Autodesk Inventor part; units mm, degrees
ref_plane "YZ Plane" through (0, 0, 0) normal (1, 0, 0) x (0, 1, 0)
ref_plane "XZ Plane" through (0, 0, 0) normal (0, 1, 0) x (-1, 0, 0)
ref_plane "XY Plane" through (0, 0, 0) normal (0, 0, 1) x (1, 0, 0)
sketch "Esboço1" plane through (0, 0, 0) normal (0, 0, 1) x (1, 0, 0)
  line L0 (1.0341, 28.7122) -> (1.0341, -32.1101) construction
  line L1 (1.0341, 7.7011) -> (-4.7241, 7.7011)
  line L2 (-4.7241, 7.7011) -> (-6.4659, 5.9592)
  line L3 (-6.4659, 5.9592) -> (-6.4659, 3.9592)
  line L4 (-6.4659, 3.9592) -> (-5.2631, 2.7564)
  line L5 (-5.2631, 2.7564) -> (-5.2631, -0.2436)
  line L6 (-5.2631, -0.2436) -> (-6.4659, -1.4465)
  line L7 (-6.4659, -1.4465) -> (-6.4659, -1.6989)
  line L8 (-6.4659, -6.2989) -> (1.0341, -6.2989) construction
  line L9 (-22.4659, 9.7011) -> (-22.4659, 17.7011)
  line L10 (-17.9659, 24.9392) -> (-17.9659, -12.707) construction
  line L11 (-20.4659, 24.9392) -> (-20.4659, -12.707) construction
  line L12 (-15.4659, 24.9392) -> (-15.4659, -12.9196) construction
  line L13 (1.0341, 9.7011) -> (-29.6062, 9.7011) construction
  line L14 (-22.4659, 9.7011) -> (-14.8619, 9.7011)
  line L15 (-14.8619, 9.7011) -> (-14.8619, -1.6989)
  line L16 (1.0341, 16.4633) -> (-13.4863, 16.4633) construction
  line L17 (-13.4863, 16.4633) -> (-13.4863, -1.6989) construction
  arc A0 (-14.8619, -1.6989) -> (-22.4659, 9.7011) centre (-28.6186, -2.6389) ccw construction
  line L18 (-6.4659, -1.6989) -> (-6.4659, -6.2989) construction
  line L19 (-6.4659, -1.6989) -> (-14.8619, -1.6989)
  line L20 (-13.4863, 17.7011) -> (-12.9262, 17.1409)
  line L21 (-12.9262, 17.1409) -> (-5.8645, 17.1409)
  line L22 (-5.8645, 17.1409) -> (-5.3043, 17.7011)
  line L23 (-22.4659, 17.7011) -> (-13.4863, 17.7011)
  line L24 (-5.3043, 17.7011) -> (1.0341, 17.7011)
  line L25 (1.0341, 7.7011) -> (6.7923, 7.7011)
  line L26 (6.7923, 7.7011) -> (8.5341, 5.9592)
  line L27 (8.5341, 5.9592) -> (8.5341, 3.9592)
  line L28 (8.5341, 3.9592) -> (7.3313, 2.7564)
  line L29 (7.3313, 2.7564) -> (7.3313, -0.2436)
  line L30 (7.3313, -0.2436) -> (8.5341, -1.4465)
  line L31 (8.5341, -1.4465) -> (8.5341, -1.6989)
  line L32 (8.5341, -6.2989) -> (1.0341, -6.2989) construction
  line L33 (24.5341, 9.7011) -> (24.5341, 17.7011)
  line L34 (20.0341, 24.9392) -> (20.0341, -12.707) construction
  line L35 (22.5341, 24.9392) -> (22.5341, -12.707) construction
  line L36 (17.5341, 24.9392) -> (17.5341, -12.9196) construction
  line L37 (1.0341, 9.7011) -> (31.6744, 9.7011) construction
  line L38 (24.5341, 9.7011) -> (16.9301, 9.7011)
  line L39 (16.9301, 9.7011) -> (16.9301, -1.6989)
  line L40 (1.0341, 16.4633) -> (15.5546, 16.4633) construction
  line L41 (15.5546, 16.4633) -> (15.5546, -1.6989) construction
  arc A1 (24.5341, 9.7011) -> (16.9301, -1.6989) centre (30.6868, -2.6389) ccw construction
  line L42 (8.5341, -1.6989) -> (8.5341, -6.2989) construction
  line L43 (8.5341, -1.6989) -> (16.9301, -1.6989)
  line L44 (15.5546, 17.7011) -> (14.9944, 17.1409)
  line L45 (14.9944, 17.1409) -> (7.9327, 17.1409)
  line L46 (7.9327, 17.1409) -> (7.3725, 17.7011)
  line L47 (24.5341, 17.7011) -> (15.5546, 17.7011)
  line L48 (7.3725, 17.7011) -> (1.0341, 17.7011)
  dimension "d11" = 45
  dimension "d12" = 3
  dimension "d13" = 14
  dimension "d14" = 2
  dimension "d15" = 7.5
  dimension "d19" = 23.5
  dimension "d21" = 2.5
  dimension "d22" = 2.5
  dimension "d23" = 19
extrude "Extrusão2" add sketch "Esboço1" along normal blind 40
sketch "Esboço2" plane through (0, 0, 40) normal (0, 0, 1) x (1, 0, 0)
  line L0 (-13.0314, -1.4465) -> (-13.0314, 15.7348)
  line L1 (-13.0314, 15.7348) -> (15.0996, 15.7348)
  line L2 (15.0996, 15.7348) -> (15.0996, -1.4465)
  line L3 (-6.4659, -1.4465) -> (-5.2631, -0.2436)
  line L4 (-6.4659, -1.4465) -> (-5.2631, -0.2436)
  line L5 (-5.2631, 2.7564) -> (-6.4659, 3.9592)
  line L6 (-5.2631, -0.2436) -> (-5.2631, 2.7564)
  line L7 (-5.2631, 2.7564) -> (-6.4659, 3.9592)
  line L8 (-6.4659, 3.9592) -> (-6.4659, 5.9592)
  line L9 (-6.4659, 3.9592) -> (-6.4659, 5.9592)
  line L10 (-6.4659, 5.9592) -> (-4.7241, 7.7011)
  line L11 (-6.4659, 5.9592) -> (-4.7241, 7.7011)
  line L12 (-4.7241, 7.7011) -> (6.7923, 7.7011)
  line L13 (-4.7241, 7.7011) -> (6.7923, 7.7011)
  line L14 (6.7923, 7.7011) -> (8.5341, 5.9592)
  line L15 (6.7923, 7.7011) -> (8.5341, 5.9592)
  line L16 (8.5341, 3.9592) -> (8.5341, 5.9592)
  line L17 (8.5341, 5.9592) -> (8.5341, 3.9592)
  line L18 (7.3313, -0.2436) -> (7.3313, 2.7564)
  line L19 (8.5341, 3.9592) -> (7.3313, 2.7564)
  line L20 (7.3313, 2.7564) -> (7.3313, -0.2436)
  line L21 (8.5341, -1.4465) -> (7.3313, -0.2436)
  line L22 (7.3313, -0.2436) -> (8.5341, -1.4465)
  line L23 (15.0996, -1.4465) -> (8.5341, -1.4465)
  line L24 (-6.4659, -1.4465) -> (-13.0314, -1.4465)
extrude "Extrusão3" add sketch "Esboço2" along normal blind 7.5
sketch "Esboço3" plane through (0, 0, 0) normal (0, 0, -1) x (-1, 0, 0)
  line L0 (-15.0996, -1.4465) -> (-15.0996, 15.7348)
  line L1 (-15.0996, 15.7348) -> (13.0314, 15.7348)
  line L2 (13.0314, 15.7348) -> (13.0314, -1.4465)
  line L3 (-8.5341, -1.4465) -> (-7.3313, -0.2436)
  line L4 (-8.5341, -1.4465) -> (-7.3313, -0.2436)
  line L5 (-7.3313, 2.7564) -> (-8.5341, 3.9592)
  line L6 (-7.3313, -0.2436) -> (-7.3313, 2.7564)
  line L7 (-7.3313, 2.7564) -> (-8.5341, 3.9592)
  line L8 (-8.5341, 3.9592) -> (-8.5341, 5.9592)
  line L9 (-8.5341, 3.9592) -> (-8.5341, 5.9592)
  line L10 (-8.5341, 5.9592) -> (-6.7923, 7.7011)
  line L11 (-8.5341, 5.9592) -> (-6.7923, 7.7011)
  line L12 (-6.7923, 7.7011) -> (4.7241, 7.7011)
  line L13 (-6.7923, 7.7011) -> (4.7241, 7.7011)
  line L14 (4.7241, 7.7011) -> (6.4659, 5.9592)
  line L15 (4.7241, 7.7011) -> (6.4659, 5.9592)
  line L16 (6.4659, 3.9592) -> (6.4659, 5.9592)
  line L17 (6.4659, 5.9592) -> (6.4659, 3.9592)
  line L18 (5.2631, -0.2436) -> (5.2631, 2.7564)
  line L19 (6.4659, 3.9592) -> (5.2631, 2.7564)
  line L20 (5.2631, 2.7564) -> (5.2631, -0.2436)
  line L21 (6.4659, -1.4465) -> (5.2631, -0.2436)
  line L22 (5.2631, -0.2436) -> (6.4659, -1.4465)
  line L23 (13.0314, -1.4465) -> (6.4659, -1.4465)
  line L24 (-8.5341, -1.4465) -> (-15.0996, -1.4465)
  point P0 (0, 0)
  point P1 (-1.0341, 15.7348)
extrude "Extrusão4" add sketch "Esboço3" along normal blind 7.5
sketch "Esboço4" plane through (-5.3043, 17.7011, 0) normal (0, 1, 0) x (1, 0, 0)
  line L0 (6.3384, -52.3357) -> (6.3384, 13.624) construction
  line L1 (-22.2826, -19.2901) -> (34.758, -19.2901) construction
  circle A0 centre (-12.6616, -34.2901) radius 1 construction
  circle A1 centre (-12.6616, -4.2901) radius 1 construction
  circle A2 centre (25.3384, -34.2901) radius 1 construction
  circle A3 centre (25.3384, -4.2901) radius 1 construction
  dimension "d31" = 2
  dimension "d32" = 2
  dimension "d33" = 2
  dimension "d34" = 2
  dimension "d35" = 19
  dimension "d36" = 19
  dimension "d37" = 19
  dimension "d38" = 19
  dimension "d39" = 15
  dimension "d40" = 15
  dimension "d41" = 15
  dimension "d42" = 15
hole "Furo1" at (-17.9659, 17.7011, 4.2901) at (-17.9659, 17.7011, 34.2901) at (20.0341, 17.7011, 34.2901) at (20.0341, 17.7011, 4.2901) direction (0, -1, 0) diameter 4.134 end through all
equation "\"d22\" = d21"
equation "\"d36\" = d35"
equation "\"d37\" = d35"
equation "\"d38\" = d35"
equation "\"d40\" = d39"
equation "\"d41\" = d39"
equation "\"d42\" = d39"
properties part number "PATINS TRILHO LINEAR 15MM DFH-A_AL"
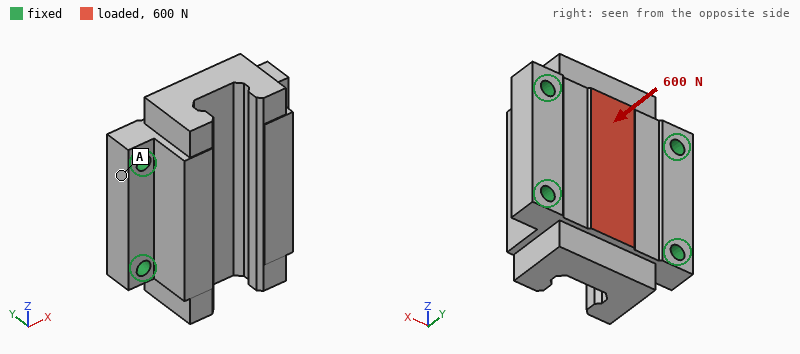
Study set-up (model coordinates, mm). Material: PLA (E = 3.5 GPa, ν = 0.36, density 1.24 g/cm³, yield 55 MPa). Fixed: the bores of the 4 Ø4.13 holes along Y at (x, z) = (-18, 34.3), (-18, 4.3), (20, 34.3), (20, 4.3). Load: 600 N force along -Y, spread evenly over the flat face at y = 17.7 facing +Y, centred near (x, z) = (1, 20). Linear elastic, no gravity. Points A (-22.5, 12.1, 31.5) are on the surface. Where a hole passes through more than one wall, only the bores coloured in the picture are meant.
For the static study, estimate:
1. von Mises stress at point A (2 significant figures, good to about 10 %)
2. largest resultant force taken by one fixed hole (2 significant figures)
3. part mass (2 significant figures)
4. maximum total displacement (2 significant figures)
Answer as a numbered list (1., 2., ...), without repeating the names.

1. 1.1 MPa
2. 160 N
3. 36 g
4. 32 µm
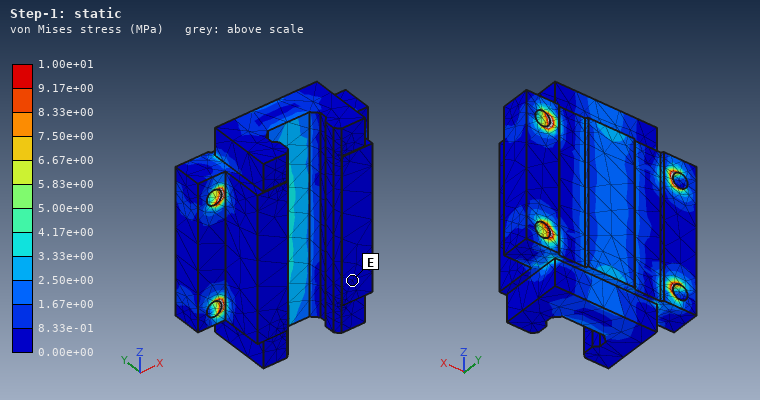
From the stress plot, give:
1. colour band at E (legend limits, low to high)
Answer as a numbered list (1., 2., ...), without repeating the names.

1. 0.00e+00 to 8.33e-01 MPa
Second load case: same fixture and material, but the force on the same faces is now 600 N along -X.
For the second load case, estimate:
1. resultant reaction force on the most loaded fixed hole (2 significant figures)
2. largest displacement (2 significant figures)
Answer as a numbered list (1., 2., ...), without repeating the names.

1. 160 N
2. 11 µm
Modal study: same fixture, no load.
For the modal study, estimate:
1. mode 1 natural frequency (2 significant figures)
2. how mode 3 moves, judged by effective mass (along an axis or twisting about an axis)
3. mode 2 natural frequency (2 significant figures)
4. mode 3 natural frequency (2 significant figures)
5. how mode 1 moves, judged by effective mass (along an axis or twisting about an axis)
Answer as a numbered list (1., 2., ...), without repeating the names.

1. 5100 Hz
2. along Z
3. 5400 Hz
4. 8400 Hz
5. along Y
